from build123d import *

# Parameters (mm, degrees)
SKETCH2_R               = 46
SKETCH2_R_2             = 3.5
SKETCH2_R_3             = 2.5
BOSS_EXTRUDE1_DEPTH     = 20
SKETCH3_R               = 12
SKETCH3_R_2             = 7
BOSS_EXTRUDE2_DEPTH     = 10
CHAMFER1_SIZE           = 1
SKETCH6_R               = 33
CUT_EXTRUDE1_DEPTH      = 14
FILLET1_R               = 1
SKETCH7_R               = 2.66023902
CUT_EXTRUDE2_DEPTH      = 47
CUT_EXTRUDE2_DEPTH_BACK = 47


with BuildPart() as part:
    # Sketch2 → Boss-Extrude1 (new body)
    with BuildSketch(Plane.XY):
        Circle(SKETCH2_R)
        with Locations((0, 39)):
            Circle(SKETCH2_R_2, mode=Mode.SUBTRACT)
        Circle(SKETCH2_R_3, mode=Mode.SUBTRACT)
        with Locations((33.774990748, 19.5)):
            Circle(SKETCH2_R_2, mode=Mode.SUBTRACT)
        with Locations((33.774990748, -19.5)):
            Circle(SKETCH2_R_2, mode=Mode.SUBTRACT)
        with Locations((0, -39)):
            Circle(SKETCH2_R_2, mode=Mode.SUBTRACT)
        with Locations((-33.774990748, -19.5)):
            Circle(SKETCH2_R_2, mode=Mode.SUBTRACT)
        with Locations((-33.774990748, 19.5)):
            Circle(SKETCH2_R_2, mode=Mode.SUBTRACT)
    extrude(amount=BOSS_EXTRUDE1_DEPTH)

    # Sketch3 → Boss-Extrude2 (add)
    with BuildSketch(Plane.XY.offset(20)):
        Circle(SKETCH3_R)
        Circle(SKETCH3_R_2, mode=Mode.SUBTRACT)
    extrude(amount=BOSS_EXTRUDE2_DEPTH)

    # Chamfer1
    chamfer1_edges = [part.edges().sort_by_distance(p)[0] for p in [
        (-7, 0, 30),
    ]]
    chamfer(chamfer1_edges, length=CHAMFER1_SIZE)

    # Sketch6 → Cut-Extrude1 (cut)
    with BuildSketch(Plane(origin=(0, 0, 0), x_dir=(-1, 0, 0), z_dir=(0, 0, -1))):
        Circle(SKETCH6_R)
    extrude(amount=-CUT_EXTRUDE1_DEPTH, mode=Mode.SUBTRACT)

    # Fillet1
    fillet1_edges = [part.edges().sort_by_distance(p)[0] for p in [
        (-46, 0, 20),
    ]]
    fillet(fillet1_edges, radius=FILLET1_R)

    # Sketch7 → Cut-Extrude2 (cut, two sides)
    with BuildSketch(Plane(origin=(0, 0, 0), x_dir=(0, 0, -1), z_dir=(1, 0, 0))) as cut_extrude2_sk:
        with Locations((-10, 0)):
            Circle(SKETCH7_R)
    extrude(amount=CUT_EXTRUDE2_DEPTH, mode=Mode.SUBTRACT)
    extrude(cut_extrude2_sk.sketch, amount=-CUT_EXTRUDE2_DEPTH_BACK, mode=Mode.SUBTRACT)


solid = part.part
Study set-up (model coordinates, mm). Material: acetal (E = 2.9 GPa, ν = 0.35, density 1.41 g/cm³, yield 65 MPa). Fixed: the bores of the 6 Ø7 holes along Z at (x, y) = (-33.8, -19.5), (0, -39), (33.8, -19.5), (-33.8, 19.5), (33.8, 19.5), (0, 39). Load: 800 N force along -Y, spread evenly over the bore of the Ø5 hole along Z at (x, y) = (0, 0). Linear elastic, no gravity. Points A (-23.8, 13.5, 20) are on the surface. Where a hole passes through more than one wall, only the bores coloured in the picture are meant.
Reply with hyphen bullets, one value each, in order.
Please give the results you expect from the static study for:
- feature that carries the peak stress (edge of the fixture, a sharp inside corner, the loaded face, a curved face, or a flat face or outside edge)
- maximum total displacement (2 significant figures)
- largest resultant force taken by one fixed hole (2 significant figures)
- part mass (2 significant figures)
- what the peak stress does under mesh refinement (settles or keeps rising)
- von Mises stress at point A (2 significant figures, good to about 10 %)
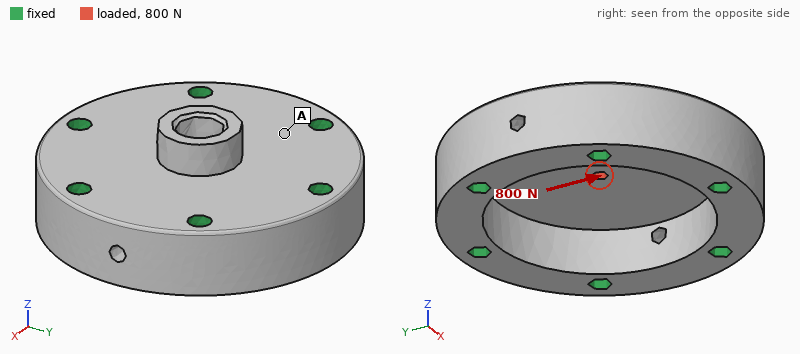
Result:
- a sharp inside corner
- 36 µm
- 210 N
- 120 g
- keeps rising
- 0.93 MPa
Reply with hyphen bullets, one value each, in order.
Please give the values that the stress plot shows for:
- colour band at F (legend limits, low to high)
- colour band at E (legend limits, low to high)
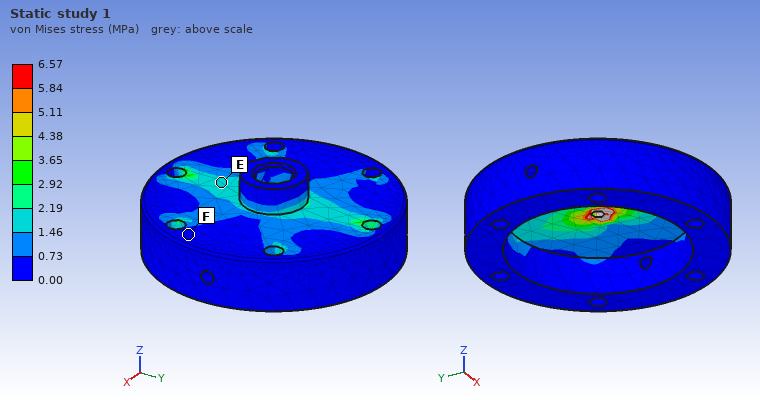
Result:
- 0.00 to 0.73 MPa
- 1.46 to 2.19 MPa
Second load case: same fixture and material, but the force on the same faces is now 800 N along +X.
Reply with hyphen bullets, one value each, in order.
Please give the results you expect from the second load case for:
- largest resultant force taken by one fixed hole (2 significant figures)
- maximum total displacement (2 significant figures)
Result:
- 180 N
- 36 µm
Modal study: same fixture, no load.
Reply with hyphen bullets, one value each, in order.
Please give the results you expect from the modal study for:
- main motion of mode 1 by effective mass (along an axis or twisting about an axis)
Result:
- along Z
